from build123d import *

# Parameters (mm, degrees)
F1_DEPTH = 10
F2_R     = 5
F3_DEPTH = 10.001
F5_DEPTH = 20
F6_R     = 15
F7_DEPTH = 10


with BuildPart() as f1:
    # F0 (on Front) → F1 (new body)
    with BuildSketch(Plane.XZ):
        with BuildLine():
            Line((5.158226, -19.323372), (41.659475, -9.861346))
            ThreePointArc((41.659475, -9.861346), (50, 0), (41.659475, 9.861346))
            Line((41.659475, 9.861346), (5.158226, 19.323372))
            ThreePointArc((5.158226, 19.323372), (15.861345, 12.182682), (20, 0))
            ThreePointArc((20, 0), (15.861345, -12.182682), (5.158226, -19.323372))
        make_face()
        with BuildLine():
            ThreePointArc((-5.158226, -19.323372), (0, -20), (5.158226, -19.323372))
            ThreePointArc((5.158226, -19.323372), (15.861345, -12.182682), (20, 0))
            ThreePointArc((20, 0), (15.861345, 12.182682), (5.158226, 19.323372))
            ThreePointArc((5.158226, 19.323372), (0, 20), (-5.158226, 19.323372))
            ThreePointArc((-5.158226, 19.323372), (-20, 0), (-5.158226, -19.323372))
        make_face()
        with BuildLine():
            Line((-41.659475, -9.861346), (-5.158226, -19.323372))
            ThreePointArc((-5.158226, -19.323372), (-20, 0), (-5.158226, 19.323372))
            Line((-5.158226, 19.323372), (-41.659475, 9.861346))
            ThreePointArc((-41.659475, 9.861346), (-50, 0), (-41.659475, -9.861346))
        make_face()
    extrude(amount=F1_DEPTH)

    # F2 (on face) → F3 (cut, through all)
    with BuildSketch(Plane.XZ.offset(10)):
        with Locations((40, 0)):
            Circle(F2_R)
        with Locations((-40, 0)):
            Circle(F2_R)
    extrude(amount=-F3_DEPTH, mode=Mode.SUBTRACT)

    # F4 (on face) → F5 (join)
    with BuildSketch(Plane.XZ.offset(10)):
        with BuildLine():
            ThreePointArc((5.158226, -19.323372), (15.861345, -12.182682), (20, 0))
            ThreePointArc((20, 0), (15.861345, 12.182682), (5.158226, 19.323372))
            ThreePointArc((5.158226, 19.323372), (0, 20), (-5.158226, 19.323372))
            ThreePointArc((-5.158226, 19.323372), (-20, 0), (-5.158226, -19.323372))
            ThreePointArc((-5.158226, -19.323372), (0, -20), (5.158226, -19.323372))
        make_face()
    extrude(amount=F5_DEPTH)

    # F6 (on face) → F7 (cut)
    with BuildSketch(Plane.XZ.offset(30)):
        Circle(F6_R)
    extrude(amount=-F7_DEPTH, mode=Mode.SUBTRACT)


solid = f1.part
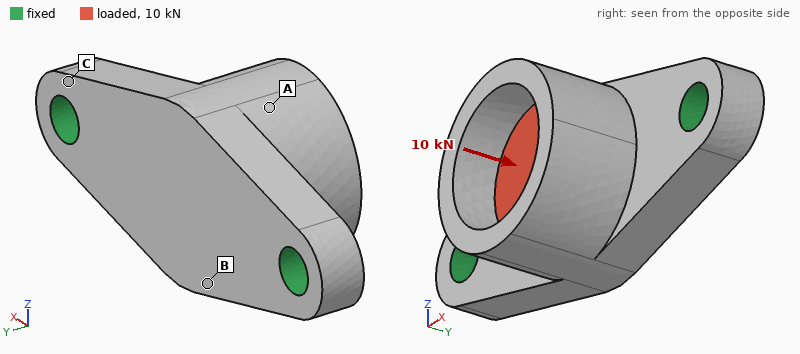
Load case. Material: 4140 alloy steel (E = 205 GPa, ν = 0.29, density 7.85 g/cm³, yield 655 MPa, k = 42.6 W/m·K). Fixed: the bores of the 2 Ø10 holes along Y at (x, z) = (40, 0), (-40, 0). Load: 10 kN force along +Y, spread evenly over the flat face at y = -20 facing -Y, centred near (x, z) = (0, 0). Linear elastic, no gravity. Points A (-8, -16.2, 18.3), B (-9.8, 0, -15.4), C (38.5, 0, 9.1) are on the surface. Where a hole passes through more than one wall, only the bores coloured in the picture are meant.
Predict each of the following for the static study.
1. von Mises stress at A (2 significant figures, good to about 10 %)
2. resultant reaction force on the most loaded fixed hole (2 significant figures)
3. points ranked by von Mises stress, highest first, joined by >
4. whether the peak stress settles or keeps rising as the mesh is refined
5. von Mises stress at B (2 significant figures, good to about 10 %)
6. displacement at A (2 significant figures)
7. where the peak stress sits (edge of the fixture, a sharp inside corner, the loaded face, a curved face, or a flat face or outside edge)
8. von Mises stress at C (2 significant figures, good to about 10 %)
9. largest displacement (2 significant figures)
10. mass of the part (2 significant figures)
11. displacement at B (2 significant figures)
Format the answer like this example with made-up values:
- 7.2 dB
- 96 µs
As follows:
- 16 MPa
- 5.5 kN
- C > B > A
- keeps rising
- 36 MPa
- 21 µm
- edge of the fixture
- 64 MPa
- 22 µm
- 350 g
- 20 µm
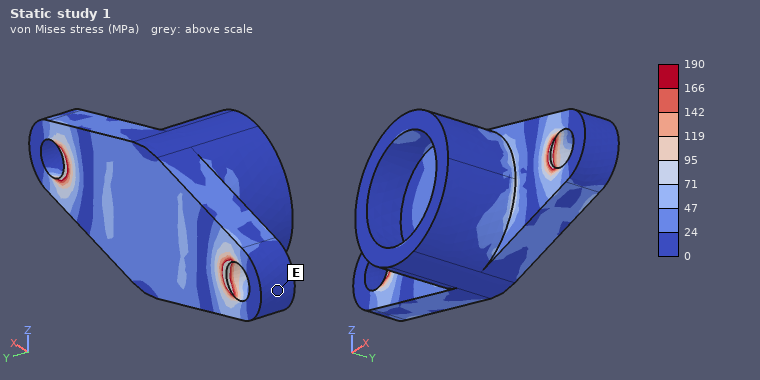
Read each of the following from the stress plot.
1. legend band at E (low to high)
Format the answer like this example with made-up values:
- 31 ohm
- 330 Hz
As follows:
- 0 to 24 MPa
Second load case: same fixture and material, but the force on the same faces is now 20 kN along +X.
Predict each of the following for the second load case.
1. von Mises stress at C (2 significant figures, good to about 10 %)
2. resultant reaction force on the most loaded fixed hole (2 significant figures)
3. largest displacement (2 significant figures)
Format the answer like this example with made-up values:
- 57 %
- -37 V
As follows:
- 66 MPa
- 11 kN
- 24 µm
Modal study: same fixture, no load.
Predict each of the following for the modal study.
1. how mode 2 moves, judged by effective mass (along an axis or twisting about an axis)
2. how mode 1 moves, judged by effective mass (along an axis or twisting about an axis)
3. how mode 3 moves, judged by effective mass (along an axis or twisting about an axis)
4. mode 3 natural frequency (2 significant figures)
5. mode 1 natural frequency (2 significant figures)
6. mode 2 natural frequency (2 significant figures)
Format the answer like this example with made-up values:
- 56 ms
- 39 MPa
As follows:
- along Y
- along Z
- along Z
- 11 kHz
- 4800 Hz
- 6900 Hz
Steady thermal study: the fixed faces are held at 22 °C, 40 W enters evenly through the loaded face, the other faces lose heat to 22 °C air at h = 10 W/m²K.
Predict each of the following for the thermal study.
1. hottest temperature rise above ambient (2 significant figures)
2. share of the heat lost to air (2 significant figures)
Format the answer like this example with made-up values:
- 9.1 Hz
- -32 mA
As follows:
- 53 K
- 7.8 %
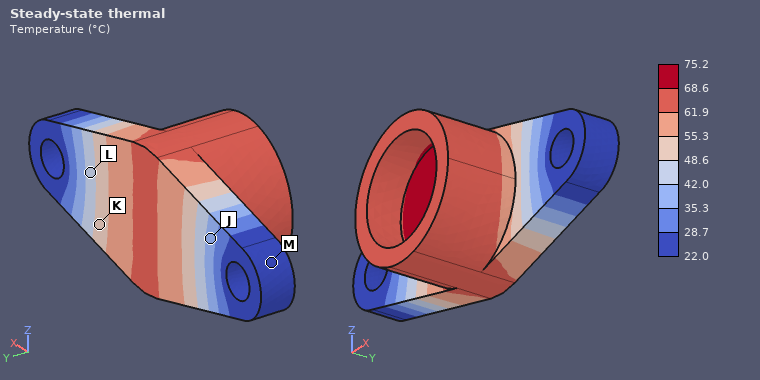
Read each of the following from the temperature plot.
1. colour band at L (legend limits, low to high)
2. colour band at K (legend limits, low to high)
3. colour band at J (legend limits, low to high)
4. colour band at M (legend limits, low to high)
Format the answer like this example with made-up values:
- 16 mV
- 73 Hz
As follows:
- 42.0 to 48.6 °C
- 48.6 to 55.3 °C
- 35.3 to 42.0 °C
- 22.0 to 28.7 °C
